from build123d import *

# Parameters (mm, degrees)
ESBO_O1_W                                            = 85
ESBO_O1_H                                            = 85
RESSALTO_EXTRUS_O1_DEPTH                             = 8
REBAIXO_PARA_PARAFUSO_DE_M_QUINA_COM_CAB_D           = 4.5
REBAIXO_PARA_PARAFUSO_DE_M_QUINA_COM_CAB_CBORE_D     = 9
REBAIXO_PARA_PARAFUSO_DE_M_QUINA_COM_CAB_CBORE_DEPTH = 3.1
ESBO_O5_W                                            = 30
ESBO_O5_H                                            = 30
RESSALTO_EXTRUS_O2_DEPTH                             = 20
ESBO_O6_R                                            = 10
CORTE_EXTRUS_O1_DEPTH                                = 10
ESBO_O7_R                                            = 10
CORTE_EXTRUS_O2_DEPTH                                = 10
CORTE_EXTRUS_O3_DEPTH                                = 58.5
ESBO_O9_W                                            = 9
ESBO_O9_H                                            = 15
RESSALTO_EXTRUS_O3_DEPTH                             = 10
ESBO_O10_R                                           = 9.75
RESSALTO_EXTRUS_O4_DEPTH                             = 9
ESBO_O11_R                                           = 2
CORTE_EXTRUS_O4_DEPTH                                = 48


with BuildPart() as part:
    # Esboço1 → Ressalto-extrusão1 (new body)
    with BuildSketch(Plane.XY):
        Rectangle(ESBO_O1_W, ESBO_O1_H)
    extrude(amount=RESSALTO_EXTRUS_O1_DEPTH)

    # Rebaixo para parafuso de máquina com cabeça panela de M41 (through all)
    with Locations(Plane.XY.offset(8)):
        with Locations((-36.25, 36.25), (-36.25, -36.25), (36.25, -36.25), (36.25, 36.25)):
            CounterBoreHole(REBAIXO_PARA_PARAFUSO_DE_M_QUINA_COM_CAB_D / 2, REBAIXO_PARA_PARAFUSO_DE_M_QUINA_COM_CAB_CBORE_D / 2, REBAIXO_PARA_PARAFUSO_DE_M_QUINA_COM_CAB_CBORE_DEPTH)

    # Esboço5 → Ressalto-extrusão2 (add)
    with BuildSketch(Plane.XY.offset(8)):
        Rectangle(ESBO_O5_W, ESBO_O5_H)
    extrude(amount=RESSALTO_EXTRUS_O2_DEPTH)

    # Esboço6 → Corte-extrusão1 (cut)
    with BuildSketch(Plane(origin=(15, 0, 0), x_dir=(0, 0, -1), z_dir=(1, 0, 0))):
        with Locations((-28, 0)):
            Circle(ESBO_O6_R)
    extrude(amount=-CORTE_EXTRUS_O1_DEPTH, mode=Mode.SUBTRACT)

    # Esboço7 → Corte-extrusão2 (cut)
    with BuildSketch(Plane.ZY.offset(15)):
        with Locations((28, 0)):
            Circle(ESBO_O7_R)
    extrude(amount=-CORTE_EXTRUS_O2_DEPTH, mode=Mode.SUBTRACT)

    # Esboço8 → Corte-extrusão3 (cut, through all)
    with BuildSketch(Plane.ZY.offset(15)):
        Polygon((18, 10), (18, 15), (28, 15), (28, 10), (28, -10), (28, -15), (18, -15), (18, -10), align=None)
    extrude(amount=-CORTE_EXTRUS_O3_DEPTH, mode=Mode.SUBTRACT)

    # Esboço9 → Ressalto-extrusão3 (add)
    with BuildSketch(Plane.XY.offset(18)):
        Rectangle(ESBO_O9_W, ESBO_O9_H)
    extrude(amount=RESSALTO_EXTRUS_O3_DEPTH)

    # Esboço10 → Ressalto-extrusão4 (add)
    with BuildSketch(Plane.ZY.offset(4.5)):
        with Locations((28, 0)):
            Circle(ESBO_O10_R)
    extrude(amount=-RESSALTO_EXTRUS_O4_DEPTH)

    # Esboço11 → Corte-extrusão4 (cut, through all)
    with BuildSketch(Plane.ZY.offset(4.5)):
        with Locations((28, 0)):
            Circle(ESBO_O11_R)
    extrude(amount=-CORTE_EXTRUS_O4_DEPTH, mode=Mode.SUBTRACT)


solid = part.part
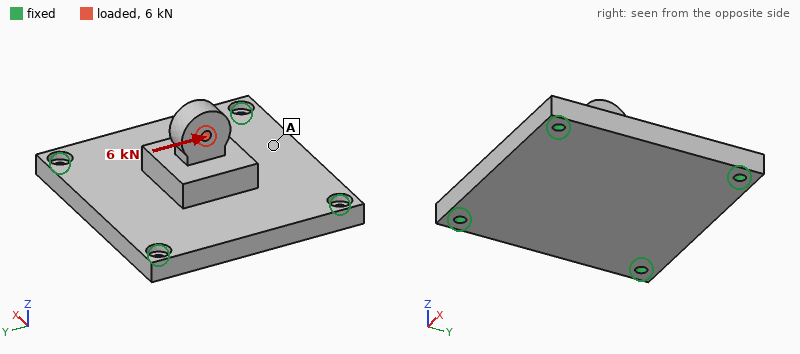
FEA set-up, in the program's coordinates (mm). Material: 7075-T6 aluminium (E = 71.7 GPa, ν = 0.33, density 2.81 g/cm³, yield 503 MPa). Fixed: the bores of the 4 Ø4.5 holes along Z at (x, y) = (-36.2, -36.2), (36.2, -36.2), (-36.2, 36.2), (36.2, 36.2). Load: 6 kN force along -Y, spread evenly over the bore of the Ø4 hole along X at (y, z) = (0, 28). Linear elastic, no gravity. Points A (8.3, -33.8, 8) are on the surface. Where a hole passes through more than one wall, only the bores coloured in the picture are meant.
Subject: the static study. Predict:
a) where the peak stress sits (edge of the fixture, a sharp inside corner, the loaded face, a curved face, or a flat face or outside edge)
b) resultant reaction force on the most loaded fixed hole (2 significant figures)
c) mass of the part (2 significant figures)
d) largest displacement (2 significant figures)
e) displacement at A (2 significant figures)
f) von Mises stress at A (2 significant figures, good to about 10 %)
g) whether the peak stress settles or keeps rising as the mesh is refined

edge of the fixture
2.3 kN
190 g
0.17 mm
0.047 mm
30 MPa
keeps rising
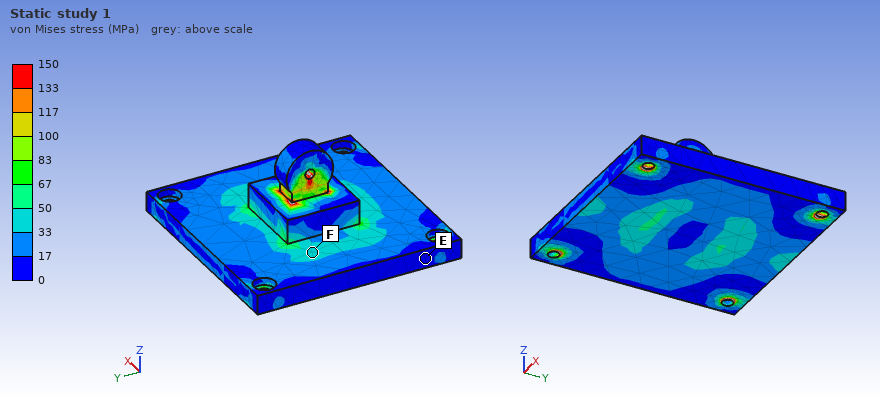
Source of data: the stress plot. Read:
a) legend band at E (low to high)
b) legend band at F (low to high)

0 to 17 MPa
33 to 50 MPa
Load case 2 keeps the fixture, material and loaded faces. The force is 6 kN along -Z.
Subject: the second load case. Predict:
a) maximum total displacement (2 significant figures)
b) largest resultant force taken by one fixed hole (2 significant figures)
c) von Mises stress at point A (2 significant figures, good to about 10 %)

0.11 mm
2.3 kN
36 MPa
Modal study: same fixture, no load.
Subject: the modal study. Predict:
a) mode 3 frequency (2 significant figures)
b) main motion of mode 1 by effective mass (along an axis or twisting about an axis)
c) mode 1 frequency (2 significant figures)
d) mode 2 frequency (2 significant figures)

6400 Hz
along Z
3800 Hz
6400 Hz
